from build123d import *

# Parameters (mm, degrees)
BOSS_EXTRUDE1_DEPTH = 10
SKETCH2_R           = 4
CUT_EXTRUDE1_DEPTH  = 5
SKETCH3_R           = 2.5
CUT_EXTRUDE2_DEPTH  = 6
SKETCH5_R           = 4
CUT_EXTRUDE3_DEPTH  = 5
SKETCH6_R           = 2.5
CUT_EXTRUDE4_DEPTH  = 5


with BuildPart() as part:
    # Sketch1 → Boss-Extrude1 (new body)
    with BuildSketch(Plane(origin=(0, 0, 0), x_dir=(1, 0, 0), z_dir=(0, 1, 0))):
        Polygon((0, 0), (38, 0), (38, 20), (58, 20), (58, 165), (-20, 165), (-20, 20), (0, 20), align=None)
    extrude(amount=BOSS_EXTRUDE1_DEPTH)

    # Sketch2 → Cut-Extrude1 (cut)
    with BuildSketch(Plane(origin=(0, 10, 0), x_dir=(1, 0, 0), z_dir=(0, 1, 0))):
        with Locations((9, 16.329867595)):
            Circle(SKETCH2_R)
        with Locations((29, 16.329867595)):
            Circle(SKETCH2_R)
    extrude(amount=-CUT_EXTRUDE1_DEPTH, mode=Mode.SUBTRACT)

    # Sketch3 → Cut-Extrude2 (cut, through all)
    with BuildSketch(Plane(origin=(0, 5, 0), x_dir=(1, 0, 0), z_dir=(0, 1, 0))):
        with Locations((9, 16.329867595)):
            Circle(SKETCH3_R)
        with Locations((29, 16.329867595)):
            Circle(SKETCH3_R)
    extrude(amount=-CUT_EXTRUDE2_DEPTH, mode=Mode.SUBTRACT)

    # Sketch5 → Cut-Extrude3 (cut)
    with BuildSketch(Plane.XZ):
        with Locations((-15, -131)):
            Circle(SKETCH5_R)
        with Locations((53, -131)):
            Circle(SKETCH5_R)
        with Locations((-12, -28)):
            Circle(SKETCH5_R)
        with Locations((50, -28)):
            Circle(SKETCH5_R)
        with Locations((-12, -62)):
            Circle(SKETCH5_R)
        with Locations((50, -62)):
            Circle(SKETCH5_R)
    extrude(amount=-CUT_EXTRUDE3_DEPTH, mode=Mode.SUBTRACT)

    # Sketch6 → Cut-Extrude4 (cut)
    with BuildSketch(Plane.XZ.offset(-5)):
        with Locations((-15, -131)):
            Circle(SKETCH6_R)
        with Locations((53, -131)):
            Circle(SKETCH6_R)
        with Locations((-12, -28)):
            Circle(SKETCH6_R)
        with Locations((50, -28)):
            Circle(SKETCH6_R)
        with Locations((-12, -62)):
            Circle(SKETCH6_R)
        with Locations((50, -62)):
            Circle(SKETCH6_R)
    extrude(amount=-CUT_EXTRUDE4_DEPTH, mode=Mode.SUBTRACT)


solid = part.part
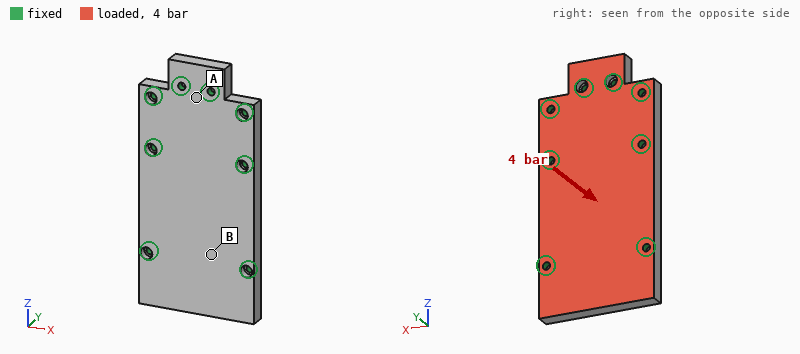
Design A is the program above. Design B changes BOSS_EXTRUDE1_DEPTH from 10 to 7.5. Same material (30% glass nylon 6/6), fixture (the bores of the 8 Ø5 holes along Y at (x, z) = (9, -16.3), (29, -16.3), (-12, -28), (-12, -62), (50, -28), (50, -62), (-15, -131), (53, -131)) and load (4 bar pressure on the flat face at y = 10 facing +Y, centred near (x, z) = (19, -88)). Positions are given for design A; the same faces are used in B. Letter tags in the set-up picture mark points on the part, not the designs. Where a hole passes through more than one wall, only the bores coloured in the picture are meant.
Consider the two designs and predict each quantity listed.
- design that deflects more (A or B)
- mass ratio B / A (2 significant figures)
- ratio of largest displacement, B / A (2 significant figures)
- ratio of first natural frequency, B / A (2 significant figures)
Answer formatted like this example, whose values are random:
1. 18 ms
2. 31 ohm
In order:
1. B
2. 0.75
3. 2.3
4. 0.76
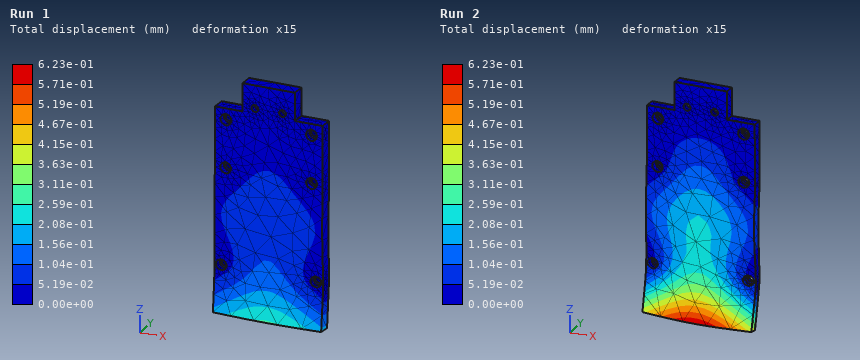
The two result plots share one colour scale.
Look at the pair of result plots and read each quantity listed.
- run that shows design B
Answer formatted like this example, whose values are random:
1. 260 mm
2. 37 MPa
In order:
1. Run 2
